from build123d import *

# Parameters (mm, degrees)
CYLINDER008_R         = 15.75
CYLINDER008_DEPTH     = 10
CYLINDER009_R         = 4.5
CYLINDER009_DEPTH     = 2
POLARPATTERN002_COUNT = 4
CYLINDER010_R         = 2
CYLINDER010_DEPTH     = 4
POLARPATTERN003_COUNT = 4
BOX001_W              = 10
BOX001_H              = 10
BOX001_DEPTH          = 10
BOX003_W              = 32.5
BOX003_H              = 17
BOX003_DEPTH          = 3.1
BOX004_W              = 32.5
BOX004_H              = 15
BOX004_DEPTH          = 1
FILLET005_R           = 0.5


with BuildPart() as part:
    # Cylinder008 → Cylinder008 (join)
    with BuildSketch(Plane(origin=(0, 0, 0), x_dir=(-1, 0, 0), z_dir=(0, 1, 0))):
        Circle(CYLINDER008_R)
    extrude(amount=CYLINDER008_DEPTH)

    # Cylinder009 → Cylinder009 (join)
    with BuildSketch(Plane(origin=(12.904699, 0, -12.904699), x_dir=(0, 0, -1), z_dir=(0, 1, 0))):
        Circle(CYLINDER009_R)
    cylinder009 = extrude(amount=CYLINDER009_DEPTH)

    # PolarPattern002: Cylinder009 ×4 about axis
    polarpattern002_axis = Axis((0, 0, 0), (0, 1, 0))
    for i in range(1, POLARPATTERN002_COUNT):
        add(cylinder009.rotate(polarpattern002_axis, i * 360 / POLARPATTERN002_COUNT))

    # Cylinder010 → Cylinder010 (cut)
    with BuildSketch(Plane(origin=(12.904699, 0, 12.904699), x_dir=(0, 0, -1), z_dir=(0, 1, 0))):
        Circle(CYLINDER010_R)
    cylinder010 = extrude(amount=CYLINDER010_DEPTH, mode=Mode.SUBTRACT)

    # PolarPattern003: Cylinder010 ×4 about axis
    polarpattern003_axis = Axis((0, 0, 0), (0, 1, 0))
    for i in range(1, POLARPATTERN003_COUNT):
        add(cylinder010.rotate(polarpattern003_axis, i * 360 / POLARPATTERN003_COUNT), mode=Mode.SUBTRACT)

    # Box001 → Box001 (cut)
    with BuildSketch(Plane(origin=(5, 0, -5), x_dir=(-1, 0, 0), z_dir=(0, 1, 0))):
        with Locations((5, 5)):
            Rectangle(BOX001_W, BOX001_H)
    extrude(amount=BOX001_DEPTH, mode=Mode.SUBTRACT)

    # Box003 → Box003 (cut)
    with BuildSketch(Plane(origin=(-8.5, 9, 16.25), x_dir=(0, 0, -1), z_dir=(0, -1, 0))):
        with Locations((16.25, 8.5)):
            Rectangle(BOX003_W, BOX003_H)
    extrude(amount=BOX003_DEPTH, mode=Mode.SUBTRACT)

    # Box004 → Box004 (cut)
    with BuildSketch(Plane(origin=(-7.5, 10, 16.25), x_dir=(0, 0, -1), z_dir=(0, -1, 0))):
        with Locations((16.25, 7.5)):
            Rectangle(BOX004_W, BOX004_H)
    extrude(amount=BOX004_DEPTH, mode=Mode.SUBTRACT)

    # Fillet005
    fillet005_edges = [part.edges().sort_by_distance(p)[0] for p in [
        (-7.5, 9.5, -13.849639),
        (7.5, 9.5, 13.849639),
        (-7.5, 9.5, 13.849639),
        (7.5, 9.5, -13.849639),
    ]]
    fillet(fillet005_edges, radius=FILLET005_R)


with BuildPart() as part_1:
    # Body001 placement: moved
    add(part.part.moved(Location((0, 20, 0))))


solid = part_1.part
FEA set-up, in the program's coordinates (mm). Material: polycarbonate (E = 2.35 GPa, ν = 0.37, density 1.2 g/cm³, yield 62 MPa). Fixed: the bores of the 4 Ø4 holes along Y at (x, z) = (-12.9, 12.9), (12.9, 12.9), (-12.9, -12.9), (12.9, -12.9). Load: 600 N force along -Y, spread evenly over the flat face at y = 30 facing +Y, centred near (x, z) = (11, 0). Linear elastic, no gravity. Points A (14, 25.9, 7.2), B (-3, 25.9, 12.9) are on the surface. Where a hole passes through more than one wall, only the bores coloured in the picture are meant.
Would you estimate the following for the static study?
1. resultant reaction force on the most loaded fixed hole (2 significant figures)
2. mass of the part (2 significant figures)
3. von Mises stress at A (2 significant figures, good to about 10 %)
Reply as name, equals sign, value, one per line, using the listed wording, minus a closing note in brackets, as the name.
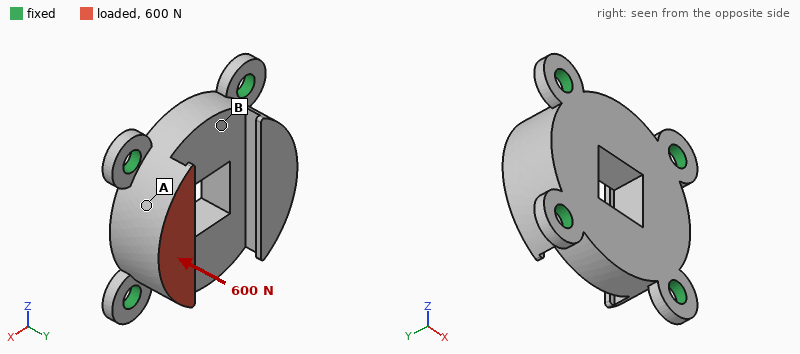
resultant reaction force on the most loaded fixed hole = 330 N
mass of the part = 6.6 g
von Mises stress at A = 9.8 MPa
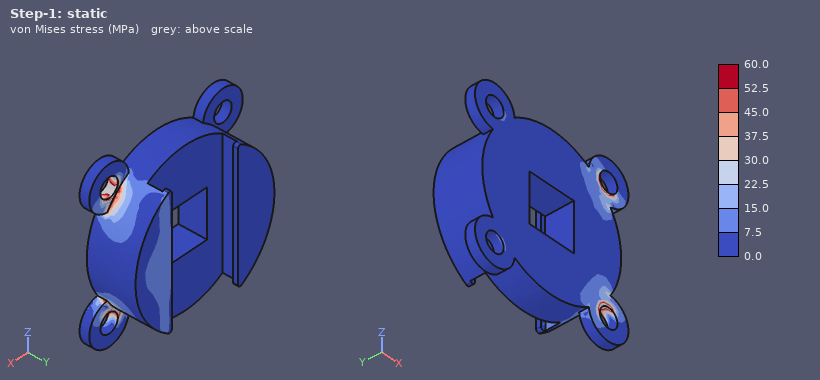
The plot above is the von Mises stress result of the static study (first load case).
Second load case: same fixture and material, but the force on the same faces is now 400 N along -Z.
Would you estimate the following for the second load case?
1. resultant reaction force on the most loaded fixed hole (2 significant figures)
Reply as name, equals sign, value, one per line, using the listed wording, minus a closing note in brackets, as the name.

resultant reaction force on the most loaded fixed hole = 230 N
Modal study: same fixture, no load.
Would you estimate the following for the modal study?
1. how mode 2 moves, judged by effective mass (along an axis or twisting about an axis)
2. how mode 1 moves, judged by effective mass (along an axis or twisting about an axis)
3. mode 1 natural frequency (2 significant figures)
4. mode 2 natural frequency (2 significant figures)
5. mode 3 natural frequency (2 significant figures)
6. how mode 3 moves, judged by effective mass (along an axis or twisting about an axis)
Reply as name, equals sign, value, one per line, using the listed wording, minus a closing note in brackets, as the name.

how mode 2 moves, judged by effective mass = along X
how mode 1 moves, judged by effective mass = along Y
mode 1 natural frequency = 5800 Hz
mode 2 natural frequency = 7000 Hz
mode 3 natural frequency = 7400 Hz
how mode 3 moves, judged by effective mass = along Y
